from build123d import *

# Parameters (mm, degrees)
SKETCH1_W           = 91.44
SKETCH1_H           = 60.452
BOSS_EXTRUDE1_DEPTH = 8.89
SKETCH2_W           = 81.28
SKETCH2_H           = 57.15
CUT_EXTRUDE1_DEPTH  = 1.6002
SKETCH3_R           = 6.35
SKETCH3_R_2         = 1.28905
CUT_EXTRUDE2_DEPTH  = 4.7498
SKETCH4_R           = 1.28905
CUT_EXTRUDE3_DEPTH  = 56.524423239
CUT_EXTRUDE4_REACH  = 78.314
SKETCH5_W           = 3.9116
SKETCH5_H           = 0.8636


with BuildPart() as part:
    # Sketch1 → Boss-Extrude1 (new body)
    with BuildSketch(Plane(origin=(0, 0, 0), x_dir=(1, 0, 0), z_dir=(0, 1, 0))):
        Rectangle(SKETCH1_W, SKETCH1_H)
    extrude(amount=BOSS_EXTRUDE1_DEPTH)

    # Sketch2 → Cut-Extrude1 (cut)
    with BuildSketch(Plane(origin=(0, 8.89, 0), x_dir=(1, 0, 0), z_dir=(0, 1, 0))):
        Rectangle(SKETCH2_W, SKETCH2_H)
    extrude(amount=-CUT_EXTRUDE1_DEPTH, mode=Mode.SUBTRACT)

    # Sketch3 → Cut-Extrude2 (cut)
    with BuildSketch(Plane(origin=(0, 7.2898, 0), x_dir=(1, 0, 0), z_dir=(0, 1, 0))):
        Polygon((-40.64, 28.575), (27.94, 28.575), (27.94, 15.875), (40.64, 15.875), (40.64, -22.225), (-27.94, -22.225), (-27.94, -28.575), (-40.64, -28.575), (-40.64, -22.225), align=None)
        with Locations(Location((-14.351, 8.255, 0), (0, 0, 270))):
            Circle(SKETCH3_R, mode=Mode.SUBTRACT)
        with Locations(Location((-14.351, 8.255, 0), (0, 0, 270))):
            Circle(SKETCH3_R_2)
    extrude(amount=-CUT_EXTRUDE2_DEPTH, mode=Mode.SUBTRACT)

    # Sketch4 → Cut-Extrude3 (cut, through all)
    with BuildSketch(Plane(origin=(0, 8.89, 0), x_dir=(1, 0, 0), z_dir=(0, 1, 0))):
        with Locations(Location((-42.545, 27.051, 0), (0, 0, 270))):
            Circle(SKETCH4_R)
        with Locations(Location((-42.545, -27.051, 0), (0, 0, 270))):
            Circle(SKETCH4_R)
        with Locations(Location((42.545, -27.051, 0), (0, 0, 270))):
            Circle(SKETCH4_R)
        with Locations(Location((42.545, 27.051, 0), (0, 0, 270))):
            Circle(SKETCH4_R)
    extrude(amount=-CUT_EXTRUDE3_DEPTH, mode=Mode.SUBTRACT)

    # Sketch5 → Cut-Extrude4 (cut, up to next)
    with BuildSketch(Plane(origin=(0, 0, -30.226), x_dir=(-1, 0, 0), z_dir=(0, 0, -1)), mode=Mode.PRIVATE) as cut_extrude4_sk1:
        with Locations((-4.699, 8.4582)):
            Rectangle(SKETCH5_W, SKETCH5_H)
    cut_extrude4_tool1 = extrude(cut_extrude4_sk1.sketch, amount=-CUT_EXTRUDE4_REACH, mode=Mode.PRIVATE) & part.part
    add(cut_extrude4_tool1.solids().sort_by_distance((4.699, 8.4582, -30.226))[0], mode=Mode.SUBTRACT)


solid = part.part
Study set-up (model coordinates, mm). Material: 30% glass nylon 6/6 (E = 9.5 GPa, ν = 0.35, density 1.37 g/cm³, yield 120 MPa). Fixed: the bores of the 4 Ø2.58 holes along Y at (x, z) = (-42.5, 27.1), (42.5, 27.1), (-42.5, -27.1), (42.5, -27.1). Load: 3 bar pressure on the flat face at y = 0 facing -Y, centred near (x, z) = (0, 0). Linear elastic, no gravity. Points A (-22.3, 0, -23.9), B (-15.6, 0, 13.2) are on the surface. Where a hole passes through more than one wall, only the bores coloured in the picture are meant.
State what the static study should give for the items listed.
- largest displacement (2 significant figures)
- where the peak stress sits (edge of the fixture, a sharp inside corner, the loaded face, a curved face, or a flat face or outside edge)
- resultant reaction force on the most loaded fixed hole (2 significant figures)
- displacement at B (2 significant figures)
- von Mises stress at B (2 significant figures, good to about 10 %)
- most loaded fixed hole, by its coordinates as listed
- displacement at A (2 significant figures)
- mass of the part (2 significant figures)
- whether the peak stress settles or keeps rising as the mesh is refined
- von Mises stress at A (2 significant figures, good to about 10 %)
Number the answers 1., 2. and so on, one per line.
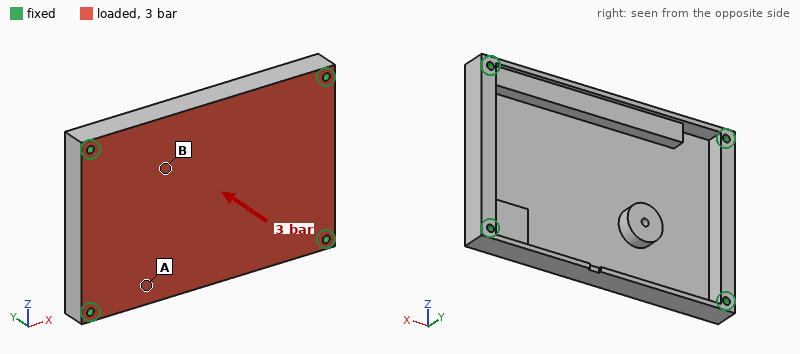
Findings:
1. 1.1 mm
2. edge of the fixture
3. 590 N
4. 0.75 mm
5. 30 MPa
6. (42.5, -27.1)
7. 0.41 mm
8. 31 g
9. keeps rising
10. 16 MPa
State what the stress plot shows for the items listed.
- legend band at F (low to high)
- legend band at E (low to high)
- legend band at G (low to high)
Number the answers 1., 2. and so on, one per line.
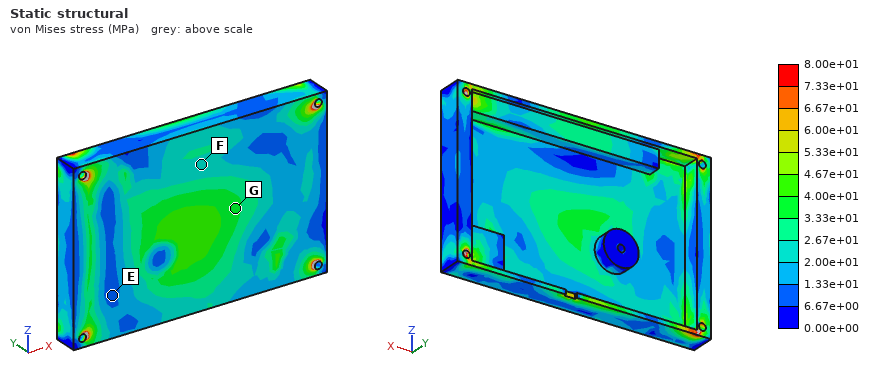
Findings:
1. 2.00e+01 to 2.67e+01 MPa
2. 6.67e+00 to 1.33e+01 MPa
3. 3.33e+01 to 4.00e+01 MPa
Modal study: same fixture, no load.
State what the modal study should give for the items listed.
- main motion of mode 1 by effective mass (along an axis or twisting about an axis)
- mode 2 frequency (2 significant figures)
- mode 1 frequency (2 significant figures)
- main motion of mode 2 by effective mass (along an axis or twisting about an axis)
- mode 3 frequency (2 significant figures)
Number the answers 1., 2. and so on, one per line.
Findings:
1. along Y
2. 2500 Hz
3. 1600 Hz
4. twisting about X
5. 3400 Hz
